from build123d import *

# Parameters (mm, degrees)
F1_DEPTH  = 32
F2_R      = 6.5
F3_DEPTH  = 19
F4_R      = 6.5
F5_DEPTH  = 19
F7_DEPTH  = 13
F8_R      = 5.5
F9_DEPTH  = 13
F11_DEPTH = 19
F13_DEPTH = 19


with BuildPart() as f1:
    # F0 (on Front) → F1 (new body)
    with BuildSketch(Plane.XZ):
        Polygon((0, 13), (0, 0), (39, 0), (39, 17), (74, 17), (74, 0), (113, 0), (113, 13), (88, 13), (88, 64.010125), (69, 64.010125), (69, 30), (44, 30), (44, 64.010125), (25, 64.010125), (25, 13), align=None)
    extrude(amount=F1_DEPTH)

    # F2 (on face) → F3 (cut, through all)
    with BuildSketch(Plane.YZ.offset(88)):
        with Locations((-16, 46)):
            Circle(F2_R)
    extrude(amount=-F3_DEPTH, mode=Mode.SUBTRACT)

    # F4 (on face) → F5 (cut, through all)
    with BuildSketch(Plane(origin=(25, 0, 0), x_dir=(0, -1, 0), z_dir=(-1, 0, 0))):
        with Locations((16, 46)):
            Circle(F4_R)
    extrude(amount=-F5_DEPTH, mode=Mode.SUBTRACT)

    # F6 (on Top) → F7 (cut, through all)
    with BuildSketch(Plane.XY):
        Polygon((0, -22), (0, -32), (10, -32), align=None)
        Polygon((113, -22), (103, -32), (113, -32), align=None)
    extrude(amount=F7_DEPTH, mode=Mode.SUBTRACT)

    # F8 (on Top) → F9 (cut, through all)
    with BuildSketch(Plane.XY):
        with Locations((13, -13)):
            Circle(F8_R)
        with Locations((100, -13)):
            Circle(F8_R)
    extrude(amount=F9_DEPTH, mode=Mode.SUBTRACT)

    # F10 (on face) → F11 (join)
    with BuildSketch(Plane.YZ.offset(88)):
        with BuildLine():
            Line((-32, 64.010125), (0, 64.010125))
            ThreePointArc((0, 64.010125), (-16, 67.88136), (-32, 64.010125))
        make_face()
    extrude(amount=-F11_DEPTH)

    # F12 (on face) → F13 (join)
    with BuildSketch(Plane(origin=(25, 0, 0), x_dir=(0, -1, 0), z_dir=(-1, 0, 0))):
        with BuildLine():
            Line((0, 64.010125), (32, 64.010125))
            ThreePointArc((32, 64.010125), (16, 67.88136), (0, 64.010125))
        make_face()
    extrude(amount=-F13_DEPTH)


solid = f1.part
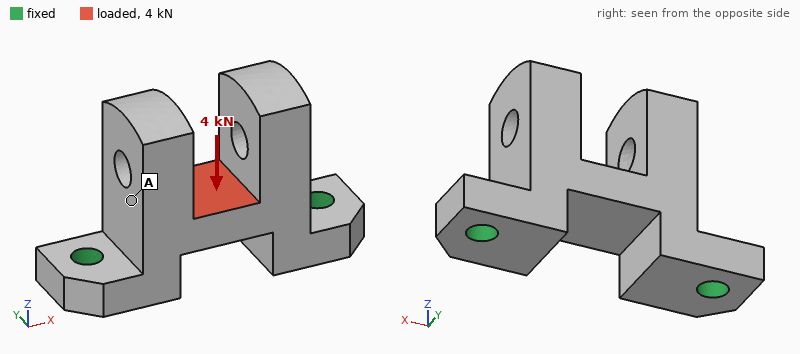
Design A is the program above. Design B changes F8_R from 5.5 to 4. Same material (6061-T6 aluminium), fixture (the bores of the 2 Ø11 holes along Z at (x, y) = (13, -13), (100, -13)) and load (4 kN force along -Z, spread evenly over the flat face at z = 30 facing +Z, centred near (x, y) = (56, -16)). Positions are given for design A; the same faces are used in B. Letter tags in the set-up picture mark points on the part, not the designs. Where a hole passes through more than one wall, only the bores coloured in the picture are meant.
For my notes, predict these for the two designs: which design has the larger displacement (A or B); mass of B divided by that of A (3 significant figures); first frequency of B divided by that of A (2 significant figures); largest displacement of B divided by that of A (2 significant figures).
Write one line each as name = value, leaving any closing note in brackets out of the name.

which design has the larger displacement = B
mass of B divided by that of A = 1.01
first frequency of B divided by that of A = 0.90
largest displacement of B divided by that of A = 1.1
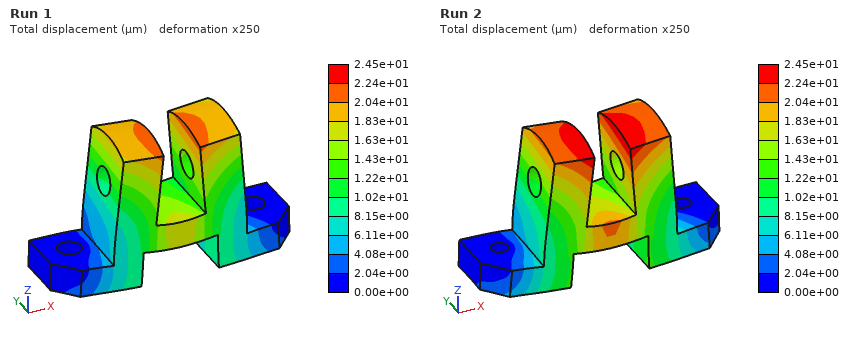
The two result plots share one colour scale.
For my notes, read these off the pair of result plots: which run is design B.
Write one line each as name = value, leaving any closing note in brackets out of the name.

which run is design B = Run 2
